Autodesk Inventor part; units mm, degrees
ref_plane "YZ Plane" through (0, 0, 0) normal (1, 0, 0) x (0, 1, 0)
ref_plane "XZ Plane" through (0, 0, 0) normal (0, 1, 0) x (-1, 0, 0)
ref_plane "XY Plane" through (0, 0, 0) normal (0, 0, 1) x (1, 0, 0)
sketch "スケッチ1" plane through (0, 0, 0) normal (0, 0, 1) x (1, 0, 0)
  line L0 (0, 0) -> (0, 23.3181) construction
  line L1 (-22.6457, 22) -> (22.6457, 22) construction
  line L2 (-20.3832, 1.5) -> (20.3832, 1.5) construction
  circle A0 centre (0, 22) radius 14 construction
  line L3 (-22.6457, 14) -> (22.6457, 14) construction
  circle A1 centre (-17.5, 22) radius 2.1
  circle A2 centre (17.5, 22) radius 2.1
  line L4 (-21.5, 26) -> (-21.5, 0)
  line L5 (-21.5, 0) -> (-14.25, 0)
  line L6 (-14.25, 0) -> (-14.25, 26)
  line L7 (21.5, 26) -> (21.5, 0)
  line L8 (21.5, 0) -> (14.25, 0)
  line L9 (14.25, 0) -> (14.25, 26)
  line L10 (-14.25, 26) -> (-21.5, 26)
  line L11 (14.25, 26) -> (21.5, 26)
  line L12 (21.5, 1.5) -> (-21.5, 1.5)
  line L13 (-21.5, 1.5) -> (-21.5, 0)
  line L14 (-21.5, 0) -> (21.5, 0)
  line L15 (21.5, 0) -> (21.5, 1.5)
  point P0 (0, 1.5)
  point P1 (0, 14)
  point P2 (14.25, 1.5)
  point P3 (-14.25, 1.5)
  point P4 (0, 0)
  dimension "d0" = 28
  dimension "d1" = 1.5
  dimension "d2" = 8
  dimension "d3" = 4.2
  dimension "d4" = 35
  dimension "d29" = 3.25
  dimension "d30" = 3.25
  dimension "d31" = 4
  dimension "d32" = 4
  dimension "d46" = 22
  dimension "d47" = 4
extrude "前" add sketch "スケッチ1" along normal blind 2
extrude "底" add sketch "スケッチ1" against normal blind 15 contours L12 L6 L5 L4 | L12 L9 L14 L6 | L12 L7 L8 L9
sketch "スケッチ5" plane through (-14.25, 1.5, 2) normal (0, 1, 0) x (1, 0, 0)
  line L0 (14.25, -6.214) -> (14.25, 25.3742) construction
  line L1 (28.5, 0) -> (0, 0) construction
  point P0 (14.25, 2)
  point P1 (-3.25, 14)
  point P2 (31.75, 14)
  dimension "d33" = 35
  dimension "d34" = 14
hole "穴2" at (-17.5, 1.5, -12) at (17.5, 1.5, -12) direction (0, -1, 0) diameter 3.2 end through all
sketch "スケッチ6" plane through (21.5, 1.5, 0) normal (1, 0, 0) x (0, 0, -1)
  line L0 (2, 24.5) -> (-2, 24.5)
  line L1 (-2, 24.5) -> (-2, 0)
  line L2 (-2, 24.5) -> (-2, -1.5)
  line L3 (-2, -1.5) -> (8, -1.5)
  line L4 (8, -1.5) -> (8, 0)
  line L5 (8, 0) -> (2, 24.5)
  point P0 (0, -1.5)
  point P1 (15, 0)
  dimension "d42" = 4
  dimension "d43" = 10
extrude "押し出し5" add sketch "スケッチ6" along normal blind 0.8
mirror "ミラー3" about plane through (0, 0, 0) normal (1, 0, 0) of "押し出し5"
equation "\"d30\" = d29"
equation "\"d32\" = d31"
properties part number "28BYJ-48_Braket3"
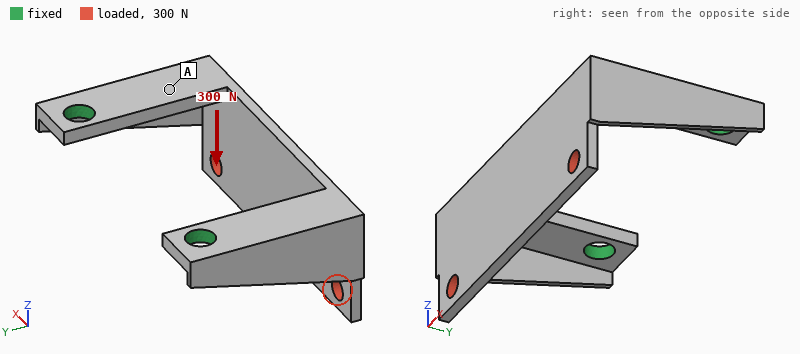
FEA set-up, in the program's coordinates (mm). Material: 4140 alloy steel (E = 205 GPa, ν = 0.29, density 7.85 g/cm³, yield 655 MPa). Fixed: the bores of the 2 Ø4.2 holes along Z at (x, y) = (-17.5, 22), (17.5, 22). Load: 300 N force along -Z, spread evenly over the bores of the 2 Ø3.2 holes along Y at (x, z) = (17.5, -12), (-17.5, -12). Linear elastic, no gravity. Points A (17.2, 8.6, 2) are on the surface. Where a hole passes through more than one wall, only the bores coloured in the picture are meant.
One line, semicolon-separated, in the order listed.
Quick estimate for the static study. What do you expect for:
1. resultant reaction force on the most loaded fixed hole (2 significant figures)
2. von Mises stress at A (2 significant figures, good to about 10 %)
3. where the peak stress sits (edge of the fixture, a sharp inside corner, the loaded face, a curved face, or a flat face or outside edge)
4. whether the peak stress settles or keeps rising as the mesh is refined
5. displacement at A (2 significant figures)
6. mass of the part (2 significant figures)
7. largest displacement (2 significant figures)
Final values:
160 N; 53 MPa; edge of the fixture; keeps rising; 0.061 mm; 16 g; 0.17 mm
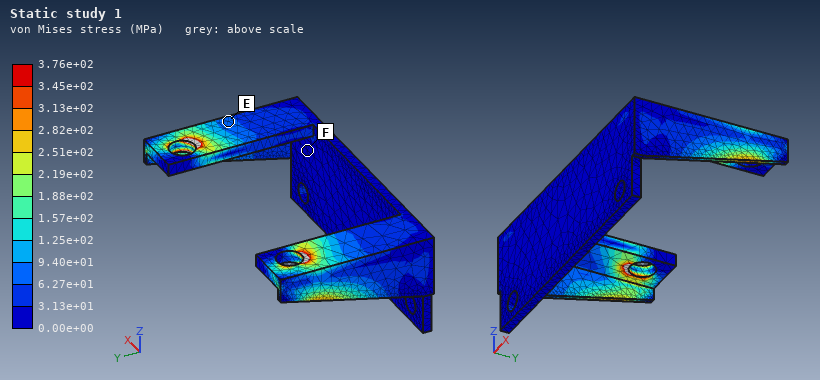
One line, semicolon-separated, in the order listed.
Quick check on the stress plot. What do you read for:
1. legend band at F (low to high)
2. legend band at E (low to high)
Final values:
0.00e+00 to 3.13e+01 MPa; 6.27e+01 to 9.40e+01 MPa
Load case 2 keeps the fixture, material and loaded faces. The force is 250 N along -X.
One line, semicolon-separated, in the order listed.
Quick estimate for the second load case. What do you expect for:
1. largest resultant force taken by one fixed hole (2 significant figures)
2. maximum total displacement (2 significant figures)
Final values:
140 N; 0.11 mm
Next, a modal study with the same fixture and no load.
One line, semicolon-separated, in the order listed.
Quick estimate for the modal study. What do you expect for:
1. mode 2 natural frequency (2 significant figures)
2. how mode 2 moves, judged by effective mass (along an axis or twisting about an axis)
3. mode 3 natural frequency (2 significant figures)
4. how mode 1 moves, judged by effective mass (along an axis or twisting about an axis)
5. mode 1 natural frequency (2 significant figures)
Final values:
3000 Hz; along X; 3900 Hz; along Z; 2200 Hz
